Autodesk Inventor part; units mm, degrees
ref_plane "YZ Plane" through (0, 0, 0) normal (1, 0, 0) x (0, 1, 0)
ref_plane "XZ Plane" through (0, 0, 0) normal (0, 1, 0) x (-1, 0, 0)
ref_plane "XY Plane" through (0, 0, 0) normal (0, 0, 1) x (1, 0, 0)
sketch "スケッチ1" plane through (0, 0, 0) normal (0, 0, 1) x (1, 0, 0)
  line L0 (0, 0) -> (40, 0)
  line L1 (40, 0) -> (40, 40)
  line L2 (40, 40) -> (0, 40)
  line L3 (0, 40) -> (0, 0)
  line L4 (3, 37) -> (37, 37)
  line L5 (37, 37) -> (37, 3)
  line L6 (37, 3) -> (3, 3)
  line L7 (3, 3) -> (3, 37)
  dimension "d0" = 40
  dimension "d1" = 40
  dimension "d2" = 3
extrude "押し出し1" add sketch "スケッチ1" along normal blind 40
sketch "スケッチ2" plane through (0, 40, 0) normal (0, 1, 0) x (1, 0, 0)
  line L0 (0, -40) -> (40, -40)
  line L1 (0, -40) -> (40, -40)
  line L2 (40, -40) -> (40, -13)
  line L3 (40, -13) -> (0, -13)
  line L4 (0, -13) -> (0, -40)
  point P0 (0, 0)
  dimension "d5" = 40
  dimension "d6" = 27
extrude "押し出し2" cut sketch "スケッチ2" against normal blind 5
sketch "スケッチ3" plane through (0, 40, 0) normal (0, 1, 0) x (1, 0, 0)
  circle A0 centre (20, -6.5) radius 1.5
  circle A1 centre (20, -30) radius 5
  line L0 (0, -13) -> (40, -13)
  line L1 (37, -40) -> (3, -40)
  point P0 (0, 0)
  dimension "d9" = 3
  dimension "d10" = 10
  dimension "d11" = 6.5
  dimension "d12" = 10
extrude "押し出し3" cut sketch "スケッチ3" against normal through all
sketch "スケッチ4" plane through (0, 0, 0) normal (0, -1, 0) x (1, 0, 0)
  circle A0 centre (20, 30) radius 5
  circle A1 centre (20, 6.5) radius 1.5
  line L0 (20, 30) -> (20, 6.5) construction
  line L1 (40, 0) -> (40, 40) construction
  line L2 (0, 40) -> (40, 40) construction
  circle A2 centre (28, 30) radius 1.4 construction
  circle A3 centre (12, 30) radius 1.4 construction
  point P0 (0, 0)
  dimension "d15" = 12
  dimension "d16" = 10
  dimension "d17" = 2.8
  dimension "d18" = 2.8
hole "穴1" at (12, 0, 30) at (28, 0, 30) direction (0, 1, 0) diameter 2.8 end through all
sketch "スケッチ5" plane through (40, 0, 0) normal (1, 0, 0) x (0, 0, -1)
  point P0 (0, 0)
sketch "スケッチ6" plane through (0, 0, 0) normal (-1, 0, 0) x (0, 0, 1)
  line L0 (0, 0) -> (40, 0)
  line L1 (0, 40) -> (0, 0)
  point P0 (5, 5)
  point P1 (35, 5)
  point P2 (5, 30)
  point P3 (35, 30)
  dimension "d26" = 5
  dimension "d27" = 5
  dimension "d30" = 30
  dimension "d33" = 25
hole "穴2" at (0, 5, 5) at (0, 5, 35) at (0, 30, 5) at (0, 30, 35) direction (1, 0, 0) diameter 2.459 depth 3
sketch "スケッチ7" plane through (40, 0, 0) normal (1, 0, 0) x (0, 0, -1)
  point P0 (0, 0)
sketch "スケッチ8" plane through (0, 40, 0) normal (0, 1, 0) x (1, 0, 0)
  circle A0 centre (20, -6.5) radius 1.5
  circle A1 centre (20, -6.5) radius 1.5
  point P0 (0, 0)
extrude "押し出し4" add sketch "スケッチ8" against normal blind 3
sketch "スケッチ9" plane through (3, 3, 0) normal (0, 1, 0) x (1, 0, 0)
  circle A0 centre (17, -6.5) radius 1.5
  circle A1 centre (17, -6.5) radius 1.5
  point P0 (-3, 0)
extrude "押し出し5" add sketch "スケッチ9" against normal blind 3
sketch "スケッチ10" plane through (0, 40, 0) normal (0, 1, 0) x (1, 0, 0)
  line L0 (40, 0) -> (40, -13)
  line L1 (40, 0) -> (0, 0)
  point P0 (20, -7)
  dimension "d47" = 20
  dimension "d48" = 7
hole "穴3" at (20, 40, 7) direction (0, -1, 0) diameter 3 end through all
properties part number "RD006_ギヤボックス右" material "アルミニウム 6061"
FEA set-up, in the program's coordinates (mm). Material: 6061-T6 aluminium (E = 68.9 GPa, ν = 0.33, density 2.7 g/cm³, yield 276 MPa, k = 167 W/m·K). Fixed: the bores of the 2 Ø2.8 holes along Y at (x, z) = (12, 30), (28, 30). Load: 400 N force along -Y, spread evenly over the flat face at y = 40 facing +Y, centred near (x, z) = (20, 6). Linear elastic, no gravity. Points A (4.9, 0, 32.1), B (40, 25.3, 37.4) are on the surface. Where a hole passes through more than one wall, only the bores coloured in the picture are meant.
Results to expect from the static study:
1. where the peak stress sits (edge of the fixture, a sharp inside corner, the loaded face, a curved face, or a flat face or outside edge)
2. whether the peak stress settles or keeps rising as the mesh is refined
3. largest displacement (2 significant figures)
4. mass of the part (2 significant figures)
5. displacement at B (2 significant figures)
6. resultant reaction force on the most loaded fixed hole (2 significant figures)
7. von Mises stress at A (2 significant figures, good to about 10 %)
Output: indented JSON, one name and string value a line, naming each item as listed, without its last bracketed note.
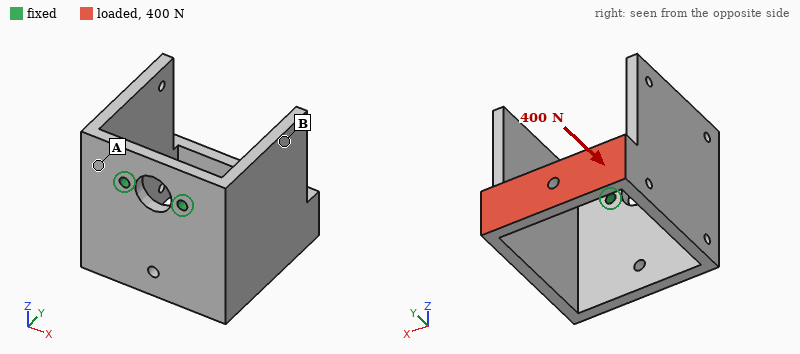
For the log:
{
  "where the peak stress sits": "edge of the fixture",
  "whether the peak stress settles or keeps rising as the mesh is refined": "keeps rising",
  "largest displacement": "0.46 mm",
  "mass of the part": "37 g",
  "displacement at B": "0.20 mm",
  "resultant reaction force on the most loaded fixed hole": "200 N",
  "von Mises stress at A": "72 MPa"
}
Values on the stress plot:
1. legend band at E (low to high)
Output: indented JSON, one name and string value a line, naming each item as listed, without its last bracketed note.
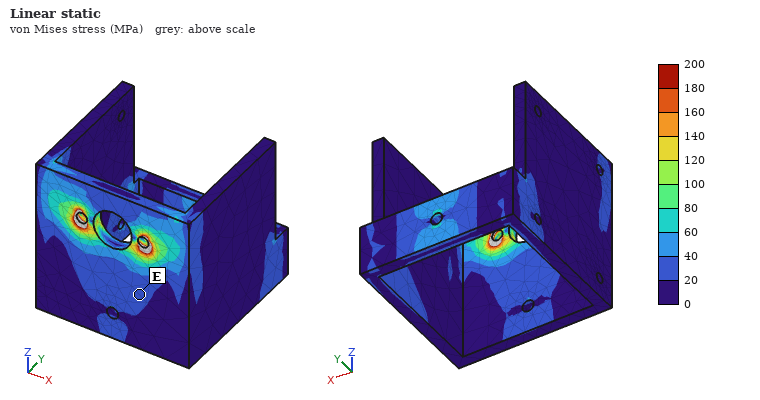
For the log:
{
  "legend band at E": "20 to 40 MPa"
}
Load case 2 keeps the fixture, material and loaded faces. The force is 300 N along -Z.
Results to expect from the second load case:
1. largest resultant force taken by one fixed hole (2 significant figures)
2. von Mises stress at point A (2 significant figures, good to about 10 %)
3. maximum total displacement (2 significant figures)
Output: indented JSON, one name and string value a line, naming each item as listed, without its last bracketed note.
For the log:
{
  "largest resultant force taken by one fixed hole": "150 N",
  "von Mises stress at point A": "86 MPa",
  "maximum total displacement": "0.53 mm"
}
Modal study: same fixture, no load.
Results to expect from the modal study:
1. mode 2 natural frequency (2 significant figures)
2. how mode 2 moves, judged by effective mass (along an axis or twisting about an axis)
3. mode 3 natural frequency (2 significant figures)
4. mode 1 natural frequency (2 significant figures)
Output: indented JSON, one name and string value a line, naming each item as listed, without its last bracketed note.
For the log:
{
  "mode 2 natural frequency": "1100 Hz",
  "how mode 2 moves, judged by effective mass": "along X",
  "mode 3 natural frequency": "2500 Hz",
  "mode 1 natural frequency": "1100 Hz"
}
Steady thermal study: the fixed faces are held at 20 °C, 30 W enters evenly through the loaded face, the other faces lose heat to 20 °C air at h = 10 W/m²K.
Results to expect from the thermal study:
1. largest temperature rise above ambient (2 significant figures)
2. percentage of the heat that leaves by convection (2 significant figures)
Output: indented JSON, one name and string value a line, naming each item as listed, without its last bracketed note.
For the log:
{
  "largest temperature rise above ambient": "80 K",
  "percentage of the heat that leaves by convection": "9.1 %"
}
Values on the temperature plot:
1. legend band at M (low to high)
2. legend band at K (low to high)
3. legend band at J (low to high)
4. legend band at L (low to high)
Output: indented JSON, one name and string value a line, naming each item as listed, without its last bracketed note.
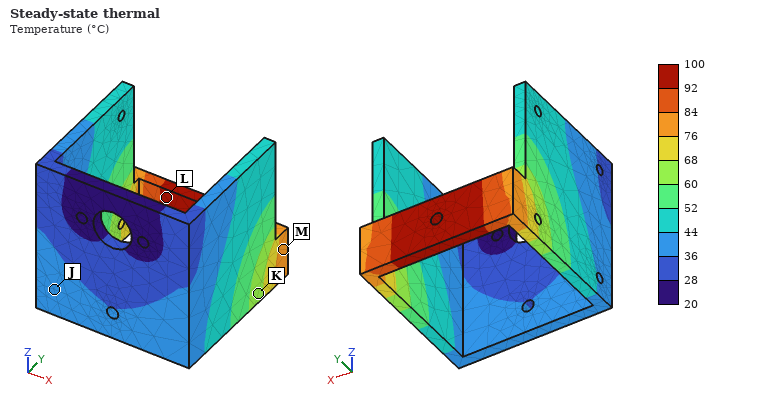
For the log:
{
  "legend band at M": "76 to 84 °C",
  "legend band at K": "60 to 68 °C",
  "legend band at J": "36 to 44 °C",
  "legend band at L": "92 to 100 °C"
}
